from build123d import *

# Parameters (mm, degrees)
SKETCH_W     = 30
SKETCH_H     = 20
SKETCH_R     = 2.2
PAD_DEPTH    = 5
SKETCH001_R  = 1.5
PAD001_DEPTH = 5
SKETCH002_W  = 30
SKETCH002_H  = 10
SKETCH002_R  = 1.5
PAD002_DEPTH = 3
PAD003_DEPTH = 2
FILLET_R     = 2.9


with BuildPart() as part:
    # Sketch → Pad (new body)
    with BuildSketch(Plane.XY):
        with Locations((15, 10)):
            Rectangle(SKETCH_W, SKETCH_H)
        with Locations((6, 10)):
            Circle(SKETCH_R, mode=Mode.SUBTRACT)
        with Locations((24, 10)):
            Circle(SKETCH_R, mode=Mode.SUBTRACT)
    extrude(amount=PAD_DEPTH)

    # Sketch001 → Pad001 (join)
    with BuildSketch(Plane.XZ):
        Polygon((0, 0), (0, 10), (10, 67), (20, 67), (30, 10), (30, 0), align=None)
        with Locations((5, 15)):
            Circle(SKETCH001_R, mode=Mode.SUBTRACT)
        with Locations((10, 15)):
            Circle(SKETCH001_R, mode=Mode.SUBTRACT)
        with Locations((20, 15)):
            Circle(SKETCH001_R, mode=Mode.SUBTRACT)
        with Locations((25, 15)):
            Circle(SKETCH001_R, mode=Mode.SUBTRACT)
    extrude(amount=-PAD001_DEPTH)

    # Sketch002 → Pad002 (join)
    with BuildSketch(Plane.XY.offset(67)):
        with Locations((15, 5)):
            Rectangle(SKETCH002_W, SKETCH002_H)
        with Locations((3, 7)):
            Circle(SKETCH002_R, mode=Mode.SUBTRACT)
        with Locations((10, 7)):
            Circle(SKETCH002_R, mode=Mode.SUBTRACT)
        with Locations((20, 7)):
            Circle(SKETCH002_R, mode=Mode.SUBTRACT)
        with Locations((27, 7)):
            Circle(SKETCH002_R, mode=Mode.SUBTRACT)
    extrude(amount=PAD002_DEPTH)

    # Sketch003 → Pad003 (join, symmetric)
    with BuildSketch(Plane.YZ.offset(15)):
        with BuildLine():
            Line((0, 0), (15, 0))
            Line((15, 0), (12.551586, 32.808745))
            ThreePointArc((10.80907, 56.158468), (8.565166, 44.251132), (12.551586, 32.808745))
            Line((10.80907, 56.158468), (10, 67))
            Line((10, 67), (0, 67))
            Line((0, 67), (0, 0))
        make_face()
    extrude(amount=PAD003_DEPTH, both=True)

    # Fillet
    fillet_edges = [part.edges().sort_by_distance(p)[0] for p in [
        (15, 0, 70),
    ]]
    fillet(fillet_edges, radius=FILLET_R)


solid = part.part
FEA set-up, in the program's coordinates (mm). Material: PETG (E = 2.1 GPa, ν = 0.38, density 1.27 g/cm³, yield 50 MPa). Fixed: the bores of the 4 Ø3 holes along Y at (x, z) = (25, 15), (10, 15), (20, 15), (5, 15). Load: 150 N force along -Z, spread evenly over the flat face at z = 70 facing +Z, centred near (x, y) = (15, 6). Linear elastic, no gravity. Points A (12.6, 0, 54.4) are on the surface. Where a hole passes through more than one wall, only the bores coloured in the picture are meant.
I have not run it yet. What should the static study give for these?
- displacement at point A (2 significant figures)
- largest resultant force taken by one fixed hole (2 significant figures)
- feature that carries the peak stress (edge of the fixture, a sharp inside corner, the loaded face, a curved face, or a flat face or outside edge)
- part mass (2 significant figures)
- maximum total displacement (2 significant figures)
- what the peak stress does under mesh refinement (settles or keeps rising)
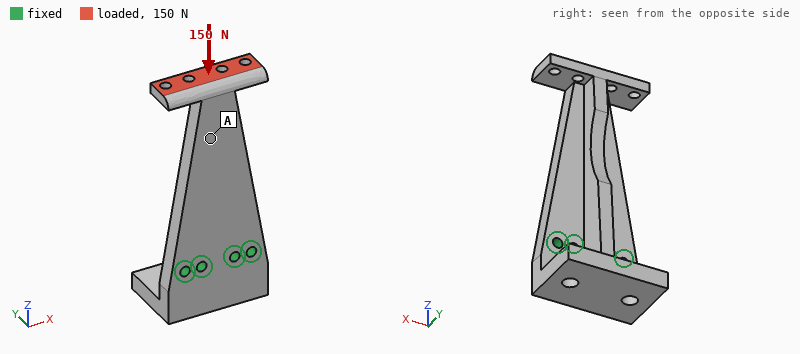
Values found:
0.24 mm
50 N
a sharp inside corner
15 g
0.87 mm
keeps rising
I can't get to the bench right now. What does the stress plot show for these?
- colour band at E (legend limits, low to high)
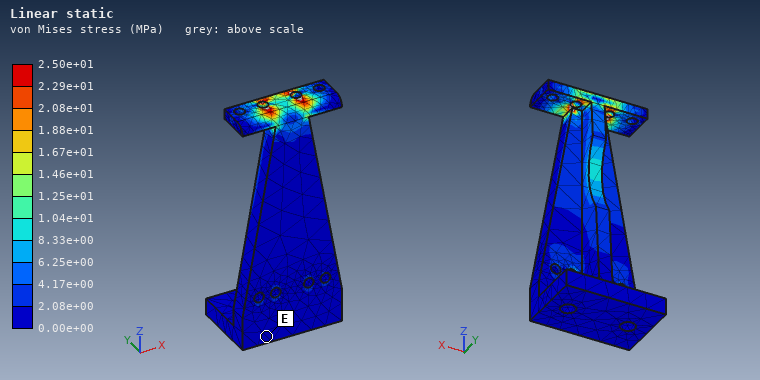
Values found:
0.00e+00 to 2.08e+00 MPa
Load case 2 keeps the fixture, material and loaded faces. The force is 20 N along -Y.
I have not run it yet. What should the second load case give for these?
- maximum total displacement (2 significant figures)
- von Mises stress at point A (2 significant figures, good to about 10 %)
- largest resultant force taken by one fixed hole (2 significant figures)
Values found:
0.76 mm
2.2 MPa
20 N
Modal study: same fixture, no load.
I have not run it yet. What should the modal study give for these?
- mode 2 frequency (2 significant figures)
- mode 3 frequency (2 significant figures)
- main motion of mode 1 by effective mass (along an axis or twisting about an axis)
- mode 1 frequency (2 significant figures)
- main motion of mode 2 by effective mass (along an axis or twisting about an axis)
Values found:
1400 Hz
1800 Hz
along Y
580 Hz
along X
